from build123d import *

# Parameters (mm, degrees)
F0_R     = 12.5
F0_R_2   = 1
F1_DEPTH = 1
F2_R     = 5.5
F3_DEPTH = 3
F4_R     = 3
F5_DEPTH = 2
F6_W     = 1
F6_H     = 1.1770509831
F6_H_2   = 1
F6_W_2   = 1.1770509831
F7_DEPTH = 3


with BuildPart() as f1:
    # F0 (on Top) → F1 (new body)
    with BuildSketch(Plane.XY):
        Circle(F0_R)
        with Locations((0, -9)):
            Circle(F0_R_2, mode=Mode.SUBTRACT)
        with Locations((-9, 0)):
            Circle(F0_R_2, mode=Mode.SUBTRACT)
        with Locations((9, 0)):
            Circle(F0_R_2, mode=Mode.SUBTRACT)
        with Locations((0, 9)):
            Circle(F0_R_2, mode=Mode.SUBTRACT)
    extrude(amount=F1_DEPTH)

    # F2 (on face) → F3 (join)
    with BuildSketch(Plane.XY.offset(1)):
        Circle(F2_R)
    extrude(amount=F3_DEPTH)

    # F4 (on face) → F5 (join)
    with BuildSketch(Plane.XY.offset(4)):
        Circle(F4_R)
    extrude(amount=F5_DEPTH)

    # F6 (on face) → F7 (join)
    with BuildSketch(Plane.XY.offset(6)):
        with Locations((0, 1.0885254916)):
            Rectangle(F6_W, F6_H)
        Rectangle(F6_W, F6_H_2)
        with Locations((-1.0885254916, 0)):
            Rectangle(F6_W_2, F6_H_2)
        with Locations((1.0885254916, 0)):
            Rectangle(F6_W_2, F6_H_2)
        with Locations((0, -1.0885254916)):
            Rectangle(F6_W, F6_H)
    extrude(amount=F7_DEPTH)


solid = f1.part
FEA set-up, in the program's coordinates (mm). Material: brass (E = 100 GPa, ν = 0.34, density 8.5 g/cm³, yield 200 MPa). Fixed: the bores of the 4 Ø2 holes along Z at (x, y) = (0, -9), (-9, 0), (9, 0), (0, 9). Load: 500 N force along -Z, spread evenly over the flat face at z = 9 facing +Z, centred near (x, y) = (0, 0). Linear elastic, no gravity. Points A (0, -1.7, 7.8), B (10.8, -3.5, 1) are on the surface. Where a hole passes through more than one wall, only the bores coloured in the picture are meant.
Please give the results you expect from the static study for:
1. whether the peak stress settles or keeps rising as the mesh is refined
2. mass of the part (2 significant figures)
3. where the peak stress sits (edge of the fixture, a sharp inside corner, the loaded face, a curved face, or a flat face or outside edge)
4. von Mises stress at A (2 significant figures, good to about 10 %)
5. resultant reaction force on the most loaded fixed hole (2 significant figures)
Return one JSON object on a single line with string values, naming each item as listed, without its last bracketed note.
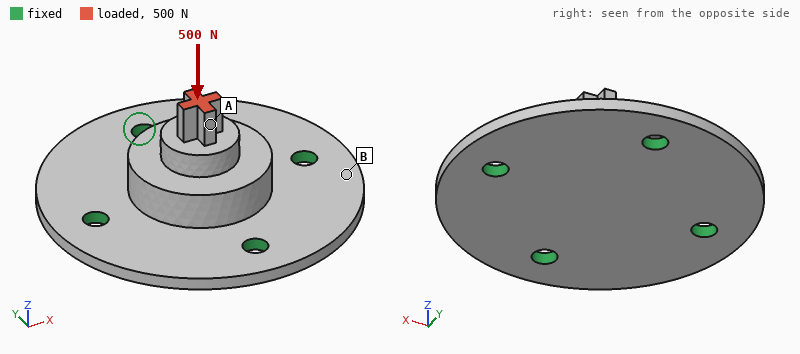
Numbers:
{"whether the peak stress settles or keeps rising as the mesh is refined": "keeps rising", "mass of the part": "7.1 g", "where the peak stress sits": "edge of the fixture", "von Mises stress at A": "85 MPa", "resultant reaction force on the most loaded fixed hole": "140 N"}
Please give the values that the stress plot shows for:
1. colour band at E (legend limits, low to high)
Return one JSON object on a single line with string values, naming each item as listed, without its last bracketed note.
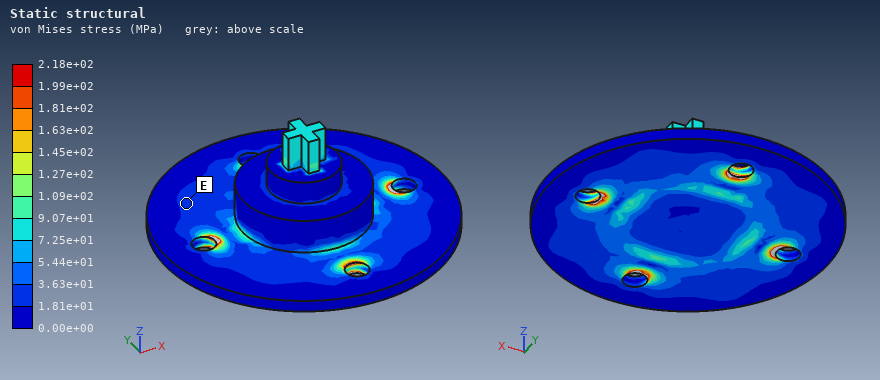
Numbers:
{"colour band at E": "1.81e+01 to 3.63e+01 MPa"}
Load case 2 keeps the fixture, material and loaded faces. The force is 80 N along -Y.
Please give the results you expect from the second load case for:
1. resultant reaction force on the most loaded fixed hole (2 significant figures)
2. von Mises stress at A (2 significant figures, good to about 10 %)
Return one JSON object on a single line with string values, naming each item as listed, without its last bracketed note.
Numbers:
{"resultant reaction force on the most loaded fixed hole": "54 N", "von Mises stress at A": "43 MPa"}
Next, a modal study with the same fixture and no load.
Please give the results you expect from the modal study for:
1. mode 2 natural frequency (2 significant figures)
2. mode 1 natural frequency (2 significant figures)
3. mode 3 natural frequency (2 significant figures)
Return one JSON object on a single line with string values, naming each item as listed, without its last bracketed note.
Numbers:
{"mode 2 natural frequency": "16 kHz", "mode 1 natural frequency": "16 kHz", "mode 3 natural frequency": "16 kHz"}
